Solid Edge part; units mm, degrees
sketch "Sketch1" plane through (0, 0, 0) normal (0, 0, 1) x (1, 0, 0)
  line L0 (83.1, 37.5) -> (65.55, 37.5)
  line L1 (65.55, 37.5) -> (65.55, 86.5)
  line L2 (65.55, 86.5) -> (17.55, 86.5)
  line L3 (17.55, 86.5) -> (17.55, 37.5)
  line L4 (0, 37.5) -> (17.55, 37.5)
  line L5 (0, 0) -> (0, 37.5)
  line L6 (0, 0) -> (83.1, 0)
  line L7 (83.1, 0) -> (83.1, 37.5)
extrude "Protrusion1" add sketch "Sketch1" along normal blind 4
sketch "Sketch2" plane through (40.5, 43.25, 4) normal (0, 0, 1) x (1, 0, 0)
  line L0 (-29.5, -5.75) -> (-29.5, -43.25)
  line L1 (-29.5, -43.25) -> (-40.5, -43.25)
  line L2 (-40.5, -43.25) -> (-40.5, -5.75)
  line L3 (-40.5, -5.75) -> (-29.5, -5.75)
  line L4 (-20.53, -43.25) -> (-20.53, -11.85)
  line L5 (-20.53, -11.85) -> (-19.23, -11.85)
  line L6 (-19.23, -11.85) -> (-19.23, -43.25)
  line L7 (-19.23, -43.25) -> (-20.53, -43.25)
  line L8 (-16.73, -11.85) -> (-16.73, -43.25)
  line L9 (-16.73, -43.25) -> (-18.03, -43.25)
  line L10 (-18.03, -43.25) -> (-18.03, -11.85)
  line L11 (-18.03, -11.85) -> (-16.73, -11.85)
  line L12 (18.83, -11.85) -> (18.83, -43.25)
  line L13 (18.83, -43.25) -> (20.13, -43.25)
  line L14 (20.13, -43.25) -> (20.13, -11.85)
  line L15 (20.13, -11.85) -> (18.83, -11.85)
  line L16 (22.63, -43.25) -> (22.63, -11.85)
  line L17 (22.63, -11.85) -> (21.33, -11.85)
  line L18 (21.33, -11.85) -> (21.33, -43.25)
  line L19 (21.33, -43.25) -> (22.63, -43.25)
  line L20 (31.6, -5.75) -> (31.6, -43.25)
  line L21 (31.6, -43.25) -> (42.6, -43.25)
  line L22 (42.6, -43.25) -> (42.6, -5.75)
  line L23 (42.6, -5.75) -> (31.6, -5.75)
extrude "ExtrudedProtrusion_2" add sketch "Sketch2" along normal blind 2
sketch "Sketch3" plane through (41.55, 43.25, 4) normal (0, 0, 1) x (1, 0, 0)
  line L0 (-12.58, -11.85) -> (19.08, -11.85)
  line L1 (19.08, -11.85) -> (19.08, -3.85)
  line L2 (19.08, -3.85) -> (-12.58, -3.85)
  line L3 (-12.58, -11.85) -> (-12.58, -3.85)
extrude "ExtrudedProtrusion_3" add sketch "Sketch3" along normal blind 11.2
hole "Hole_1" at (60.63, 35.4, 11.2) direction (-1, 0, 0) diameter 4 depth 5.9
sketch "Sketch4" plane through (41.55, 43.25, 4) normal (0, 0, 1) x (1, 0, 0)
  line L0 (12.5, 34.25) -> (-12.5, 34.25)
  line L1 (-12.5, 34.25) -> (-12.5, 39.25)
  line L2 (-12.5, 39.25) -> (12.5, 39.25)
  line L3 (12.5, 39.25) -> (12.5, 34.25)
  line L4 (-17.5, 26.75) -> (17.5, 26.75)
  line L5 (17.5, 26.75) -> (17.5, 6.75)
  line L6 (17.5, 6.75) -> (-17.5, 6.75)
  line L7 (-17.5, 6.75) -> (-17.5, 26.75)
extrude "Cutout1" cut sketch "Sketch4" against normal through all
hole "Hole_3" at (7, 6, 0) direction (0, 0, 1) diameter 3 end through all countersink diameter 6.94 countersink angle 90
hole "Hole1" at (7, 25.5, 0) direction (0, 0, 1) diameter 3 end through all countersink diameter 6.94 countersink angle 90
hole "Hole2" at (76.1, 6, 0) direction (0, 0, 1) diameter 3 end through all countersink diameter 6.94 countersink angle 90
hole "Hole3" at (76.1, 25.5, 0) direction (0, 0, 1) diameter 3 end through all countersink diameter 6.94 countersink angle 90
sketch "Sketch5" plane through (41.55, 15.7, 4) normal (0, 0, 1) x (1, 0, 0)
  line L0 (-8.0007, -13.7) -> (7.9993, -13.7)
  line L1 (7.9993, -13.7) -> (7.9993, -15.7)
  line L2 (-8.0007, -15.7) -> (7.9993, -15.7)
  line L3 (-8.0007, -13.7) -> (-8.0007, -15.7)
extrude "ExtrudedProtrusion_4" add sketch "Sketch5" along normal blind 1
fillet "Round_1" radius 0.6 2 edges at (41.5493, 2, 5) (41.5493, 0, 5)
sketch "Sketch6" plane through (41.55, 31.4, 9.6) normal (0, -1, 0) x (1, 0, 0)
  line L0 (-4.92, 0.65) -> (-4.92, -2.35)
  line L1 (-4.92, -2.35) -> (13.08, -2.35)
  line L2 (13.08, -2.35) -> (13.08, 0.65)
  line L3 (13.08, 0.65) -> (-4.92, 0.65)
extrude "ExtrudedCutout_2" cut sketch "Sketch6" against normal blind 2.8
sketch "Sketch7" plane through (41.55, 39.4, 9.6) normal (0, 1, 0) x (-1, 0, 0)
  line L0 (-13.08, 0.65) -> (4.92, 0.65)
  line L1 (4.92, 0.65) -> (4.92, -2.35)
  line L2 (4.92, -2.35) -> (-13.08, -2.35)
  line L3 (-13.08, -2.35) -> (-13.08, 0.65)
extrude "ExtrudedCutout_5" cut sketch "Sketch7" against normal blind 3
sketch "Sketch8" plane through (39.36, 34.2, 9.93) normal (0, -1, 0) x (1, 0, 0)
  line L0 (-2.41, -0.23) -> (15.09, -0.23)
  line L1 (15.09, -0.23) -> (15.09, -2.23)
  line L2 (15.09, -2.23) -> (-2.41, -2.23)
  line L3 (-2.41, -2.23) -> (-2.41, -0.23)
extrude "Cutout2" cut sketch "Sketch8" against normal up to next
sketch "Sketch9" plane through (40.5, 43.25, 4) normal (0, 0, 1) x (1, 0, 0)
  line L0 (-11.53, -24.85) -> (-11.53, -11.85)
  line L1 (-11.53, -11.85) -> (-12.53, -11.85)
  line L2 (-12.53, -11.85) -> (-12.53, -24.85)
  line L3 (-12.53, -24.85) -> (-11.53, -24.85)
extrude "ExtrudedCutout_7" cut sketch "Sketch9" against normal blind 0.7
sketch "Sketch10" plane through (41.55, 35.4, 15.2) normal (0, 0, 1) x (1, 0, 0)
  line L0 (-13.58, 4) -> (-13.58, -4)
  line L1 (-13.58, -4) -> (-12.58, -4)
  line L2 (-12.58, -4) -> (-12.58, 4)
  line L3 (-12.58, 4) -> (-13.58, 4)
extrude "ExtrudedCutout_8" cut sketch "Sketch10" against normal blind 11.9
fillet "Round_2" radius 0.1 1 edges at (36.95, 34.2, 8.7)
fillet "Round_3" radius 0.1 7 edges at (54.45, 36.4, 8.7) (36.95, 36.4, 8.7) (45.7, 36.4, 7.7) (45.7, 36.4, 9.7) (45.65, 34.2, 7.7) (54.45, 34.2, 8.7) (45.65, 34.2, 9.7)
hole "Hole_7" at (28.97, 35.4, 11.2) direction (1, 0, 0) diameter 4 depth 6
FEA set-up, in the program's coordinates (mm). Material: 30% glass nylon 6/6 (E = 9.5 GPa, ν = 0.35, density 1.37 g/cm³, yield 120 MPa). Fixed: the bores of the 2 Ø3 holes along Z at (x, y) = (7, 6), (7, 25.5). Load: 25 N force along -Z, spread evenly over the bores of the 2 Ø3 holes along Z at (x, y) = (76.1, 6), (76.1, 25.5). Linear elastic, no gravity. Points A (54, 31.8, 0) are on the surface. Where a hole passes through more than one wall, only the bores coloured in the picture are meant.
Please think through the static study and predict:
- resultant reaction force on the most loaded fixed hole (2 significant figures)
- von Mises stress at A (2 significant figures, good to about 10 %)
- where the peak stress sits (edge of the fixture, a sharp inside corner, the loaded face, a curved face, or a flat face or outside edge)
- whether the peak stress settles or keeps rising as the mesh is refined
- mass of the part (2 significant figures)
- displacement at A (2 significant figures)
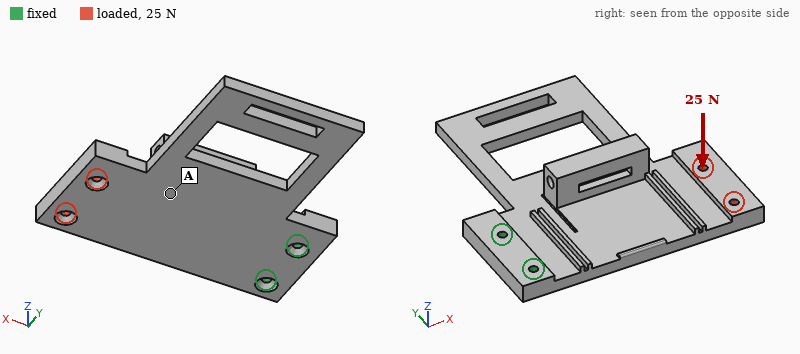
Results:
22 N
2.3 MPa
edge of the fixture
keeps rising
31 g
0.65 mm
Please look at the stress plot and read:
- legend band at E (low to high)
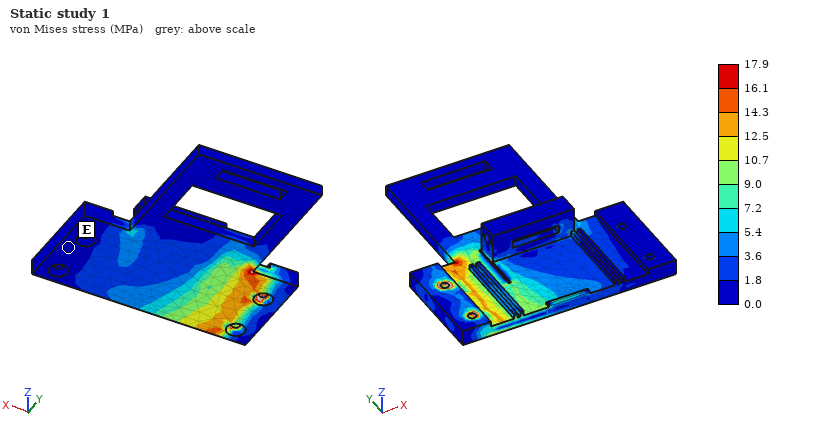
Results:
0.0 to 1.8 MPa
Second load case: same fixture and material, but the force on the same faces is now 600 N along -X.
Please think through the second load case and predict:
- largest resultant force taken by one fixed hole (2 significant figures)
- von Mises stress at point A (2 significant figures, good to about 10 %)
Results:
300 N
2.6 MPa
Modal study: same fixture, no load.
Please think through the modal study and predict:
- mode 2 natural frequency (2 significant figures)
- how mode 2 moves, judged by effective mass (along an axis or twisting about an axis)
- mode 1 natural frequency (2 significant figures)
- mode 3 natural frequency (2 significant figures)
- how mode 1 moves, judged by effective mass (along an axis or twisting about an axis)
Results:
390 Hz
twisting about X
240 Hz
1100 Hz
along Z
